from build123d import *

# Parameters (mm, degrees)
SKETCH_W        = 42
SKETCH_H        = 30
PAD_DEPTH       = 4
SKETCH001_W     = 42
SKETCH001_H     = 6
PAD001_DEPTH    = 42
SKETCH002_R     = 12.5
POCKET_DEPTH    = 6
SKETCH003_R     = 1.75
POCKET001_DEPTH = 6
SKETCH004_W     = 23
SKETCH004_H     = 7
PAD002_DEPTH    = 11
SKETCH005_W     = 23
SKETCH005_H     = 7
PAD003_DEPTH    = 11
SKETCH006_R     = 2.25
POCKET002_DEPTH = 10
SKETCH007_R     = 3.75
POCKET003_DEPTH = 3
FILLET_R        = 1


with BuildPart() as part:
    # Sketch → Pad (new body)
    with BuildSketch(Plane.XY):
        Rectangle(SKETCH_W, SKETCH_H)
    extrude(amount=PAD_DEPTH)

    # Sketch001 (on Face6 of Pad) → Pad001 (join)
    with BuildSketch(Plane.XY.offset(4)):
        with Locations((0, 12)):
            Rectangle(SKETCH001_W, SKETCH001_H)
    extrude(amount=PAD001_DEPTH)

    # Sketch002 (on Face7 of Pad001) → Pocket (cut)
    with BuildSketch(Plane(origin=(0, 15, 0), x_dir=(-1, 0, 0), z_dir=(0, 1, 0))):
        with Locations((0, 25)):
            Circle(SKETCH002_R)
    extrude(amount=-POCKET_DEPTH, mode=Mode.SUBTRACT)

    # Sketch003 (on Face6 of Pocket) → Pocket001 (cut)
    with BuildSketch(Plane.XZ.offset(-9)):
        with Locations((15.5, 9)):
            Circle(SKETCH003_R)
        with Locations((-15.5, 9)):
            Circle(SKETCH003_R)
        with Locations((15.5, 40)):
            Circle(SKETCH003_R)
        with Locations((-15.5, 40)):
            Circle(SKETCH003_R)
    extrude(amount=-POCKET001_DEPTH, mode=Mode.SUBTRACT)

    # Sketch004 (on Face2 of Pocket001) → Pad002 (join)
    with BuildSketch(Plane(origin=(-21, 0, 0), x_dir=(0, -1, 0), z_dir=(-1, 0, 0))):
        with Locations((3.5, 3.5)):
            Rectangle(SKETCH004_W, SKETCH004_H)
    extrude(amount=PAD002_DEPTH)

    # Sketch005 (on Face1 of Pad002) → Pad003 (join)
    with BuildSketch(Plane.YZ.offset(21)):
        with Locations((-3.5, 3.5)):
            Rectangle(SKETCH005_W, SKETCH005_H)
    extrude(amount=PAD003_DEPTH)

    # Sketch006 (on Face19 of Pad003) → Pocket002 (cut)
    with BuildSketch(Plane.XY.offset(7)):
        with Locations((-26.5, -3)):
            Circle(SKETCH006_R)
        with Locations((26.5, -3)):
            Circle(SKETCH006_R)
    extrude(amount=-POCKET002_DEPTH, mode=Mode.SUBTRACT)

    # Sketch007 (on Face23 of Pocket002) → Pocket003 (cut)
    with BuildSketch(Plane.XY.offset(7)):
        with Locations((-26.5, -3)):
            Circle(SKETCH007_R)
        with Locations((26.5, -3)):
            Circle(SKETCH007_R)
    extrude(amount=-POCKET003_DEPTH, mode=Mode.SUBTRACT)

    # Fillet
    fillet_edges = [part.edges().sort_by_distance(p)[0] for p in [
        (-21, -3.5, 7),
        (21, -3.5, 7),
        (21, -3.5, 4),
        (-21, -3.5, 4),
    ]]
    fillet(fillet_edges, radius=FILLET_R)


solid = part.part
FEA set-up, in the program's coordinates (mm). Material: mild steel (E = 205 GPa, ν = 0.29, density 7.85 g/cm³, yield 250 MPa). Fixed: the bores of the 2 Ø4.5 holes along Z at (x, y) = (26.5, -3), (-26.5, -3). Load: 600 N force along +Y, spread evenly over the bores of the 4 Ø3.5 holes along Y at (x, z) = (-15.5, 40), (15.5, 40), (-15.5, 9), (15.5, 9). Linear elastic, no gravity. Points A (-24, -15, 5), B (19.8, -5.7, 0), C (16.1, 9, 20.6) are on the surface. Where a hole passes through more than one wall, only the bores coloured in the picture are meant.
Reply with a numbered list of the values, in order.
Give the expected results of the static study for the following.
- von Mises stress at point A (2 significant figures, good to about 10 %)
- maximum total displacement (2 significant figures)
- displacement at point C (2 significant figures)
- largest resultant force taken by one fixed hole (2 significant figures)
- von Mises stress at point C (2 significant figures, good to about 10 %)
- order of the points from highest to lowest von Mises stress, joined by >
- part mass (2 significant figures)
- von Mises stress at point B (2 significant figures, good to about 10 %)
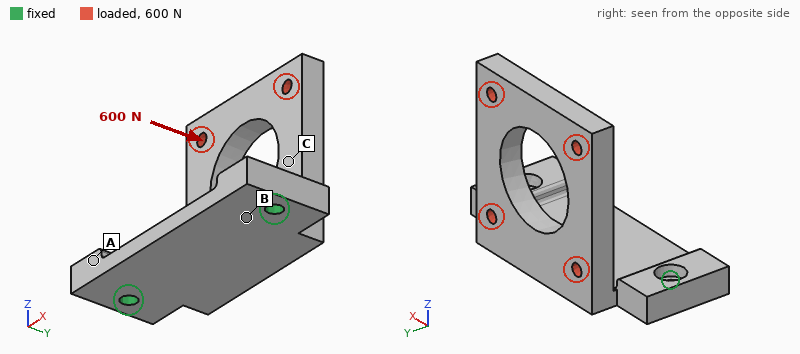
1. 15 MPa
2. 0.24 mm
3. 0.083 mm
4. 320 N
5. 49 MPa
6. C > B > A
7. 120 g
8. 27 MPa
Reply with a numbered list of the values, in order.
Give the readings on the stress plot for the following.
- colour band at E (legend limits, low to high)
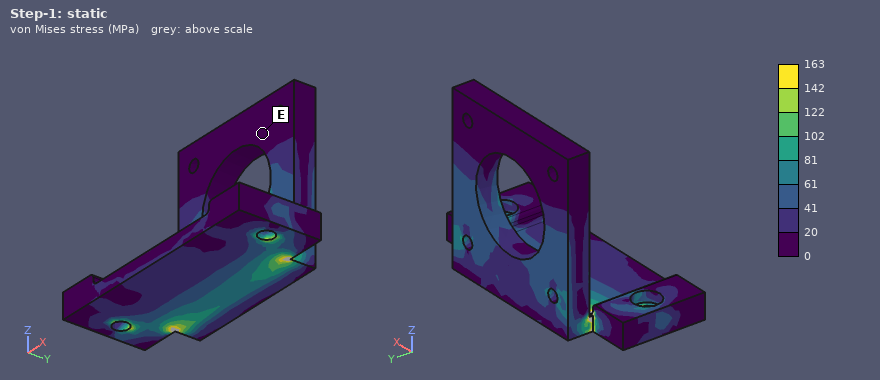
1. 0 to 20 MPa
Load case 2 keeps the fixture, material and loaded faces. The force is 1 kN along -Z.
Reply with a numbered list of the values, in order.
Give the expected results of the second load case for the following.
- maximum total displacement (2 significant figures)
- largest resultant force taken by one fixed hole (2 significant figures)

1. 99 µm
2. 500 N
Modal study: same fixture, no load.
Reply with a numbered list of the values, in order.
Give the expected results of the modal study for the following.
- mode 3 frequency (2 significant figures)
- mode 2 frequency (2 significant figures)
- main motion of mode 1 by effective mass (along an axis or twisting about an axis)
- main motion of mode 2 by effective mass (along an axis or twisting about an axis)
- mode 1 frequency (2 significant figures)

1. 4700 Hz
2. 3300 Hz
3. along Y
4. along X
5. 1200 Hz
